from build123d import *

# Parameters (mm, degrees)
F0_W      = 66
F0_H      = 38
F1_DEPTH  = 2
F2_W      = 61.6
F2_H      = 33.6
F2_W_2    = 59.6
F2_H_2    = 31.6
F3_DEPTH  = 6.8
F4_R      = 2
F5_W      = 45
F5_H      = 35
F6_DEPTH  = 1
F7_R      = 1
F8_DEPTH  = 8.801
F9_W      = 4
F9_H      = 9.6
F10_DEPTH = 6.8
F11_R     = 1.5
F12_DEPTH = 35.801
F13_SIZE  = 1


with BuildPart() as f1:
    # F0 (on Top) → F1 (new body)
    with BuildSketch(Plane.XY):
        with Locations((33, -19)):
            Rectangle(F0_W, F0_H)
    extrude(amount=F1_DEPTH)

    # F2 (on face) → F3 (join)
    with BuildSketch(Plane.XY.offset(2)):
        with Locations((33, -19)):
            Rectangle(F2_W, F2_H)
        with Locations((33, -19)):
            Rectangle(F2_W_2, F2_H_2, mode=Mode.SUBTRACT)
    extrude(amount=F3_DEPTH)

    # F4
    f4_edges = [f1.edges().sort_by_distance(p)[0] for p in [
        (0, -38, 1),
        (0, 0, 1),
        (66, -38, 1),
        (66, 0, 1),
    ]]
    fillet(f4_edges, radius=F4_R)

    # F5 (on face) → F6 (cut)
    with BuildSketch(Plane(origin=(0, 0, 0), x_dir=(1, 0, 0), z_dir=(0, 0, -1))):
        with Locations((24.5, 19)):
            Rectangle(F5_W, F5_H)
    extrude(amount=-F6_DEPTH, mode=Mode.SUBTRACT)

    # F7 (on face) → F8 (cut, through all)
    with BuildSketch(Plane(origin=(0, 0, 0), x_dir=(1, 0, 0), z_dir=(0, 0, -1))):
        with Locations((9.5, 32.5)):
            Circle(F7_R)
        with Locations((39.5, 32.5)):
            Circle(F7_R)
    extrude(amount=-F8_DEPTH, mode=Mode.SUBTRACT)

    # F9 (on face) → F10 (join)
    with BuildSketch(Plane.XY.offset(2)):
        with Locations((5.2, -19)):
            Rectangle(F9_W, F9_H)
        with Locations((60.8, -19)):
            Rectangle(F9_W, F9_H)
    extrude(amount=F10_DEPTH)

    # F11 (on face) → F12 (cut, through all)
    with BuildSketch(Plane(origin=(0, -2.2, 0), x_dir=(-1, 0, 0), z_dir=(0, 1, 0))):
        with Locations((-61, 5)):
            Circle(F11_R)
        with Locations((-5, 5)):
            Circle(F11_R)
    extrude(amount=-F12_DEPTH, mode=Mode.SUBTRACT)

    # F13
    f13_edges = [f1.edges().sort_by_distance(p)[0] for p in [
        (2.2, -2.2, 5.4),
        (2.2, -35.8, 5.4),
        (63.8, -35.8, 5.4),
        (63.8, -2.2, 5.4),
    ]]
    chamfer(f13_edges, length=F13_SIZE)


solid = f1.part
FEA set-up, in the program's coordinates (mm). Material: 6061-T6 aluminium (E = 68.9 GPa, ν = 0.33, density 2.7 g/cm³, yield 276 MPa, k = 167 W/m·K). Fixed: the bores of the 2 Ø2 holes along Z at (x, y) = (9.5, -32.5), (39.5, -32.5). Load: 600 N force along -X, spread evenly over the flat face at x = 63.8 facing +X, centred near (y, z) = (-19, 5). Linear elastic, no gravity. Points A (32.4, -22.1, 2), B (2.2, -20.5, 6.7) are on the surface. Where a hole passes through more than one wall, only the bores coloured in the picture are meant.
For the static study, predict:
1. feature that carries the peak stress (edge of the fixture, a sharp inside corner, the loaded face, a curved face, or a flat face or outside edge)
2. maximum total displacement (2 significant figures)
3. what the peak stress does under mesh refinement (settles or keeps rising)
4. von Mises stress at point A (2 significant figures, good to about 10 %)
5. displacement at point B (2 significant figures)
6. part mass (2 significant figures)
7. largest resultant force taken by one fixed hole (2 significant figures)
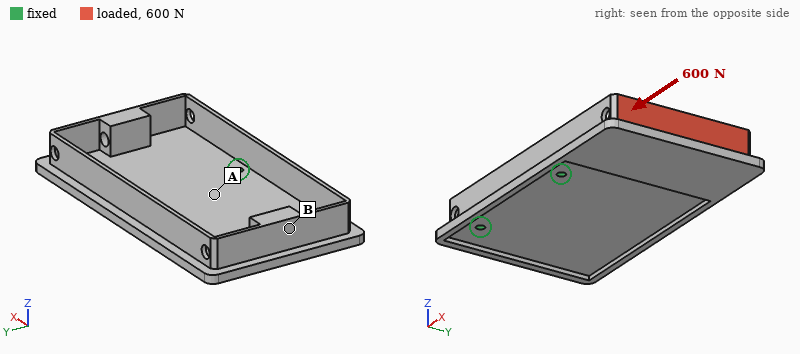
edge of the fixture
0.64 mm
keeps rising
40 MPa
0.10 mm
14 g
410 N
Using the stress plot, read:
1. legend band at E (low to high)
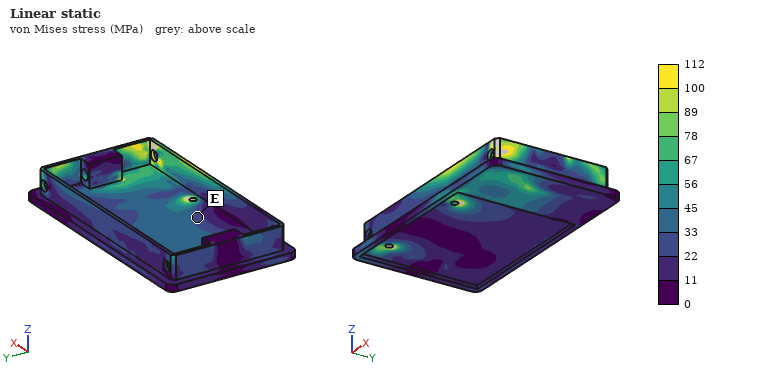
22 to 33 MPa
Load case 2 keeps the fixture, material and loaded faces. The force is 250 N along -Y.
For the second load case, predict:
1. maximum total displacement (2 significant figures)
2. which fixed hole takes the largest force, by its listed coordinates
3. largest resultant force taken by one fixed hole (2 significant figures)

0.92 mm
(39.5, -32.5)
450 N
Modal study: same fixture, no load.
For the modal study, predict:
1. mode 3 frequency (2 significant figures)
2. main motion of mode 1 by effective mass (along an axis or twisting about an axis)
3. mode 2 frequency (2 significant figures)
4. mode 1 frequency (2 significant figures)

3700 Hz
along Z
1200 Hz
590 Hz
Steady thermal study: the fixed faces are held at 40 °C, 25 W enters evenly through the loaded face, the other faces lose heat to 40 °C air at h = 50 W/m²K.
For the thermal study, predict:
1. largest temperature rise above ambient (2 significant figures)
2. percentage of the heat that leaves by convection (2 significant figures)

74 K
43 %
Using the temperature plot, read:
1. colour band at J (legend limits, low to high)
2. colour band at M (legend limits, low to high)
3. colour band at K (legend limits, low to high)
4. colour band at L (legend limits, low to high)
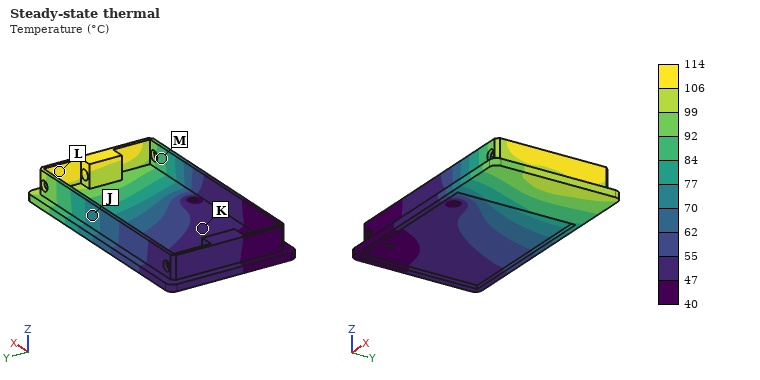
70 to 77 °C
84 to 92 °C
47 to 55 °C
106 to 114 °C
